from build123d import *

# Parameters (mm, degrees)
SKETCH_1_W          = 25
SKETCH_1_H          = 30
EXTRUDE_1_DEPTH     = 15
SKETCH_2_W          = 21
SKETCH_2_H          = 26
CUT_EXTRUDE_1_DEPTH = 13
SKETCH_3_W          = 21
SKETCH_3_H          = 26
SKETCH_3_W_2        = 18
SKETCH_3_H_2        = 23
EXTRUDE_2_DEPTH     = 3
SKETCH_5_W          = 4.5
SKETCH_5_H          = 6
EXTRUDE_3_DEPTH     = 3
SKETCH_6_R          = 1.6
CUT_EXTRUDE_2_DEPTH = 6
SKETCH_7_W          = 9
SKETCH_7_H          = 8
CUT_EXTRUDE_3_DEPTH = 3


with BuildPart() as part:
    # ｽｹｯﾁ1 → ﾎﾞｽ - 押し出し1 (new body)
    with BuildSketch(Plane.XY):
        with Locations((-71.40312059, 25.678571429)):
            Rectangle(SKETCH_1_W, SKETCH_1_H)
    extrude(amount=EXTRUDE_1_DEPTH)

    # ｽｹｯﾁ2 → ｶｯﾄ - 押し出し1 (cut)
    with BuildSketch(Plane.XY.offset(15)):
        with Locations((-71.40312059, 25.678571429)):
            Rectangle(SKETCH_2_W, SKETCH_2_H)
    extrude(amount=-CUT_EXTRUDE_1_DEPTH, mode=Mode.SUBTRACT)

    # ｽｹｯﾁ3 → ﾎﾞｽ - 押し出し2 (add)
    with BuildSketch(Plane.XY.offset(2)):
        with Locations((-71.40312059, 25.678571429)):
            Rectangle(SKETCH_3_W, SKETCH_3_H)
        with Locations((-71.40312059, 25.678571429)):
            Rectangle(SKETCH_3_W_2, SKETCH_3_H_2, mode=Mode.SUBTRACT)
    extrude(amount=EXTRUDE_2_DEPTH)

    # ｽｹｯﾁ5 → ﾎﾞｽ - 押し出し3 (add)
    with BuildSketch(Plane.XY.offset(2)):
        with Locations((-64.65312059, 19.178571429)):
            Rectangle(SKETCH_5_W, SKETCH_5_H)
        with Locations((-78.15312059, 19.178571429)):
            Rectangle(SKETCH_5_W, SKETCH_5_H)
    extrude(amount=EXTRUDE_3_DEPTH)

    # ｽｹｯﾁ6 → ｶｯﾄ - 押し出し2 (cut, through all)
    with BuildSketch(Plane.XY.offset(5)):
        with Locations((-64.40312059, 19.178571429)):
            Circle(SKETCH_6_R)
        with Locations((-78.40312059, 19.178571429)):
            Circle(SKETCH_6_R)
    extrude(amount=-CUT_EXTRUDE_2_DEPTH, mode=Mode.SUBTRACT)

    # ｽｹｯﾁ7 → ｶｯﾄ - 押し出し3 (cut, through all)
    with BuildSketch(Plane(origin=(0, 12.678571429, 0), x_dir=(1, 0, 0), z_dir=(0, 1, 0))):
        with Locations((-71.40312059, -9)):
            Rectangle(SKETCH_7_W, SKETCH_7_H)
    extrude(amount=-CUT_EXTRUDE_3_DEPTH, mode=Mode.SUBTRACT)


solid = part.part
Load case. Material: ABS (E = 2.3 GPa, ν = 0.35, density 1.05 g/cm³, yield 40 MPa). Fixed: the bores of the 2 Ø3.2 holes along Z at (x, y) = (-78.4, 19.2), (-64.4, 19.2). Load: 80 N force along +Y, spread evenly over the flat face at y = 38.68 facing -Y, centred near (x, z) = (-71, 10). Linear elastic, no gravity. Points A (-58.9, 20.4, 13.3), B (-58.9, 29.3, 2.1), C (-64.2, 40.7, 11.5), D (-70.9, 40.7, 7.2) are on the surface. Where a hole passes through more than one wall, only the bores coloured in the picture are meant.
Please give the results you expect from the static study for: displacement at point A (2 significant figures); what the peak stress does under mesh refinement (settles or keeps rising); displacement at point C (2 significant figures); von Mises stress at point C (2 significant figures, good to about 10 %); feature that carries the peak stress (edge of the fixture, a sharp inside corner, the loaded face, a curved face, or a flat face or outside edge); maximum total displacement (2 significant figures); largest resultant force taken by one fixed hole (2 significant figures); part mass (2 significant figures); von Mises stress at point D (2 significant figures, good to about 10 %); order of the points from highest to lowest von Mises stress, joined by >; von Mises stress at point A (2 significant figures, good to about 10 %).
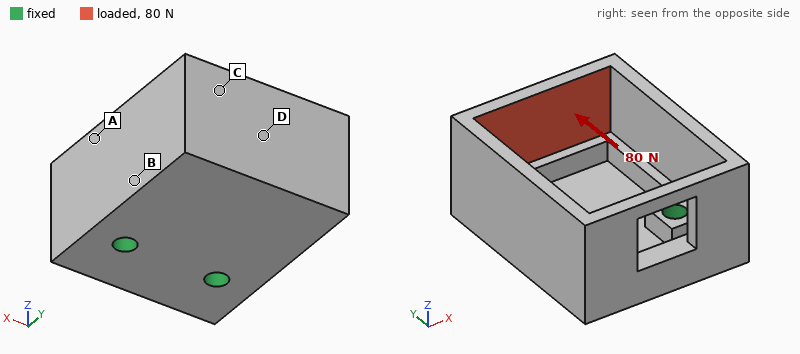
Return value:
0.070 mm
keeps rising
0.21 mm
7.2 MPa
edge of the fixture
0.36 mm
40 N
4.7 g
4.9 MPa
C > D > A > B
2.4 MPa
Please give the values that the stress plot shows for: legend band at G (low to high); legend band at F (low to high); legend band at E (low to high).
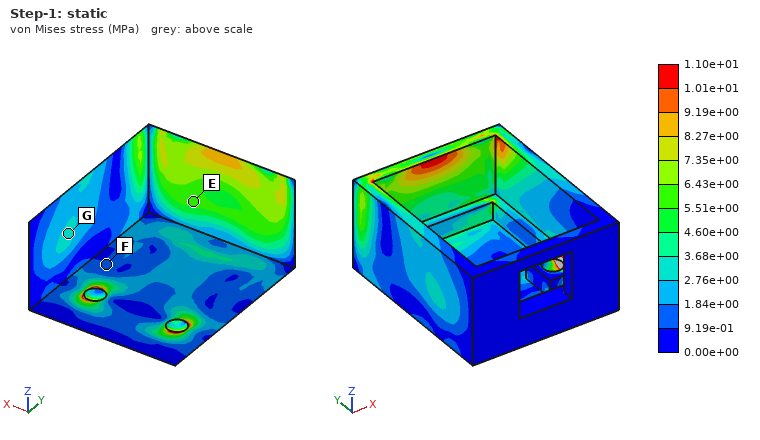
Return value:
2.76e+00 to 3.68e+00 MPa
9.19e-01 to 1.84e+00 MPa
5.51e+00 to 6.43e+00 MPa
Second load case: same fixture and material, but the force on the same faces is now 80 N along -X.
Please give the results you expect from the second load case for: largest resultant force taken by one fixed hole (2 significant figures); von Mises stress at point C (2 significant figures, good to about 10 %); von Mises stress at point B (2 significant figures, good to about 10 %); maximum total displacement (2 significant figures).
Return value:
100 N
3.6 MPa
5.6 MPa
0.44 mm
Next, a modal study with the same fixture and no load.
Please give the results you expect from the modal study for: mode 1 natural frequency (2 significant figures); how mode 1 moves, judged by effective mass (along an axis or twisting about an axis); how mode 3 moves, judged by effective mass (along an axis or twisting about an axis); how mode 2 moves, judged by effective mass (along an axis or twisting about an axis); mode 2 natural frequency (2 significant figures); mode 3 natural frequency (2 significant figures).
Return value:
1800 Hz
along Z
along X
along X
2100 Hz
4500 Hz
